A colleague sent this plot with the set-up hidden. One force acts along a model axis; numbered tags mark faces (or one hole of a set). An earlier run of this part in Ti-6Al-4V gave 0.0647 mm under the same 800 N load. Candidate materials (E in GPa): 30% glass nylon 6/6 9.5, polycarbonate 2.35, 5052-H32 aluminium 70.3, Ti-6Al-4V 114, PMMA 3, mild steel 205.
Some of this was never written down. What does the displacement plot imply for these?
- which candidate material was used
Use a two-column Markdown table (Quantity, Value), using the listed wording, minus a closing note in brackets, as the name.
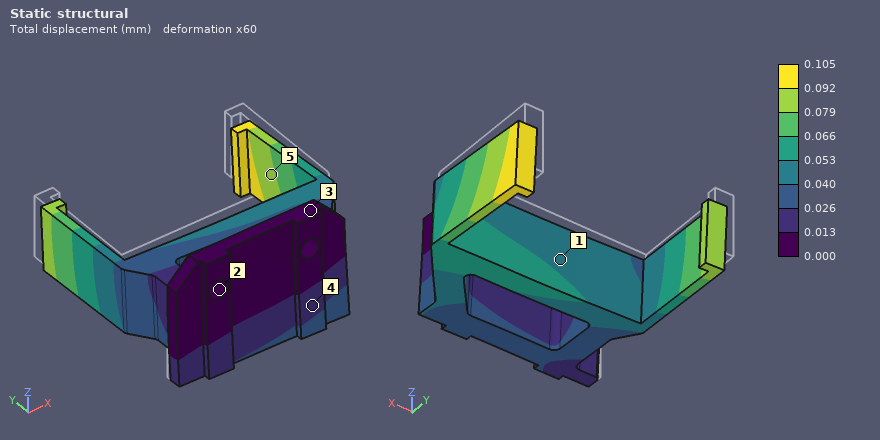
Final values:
| Quantity | Value |
|---|---|
| which candidate material was used | 5052-H32 aluminium |
